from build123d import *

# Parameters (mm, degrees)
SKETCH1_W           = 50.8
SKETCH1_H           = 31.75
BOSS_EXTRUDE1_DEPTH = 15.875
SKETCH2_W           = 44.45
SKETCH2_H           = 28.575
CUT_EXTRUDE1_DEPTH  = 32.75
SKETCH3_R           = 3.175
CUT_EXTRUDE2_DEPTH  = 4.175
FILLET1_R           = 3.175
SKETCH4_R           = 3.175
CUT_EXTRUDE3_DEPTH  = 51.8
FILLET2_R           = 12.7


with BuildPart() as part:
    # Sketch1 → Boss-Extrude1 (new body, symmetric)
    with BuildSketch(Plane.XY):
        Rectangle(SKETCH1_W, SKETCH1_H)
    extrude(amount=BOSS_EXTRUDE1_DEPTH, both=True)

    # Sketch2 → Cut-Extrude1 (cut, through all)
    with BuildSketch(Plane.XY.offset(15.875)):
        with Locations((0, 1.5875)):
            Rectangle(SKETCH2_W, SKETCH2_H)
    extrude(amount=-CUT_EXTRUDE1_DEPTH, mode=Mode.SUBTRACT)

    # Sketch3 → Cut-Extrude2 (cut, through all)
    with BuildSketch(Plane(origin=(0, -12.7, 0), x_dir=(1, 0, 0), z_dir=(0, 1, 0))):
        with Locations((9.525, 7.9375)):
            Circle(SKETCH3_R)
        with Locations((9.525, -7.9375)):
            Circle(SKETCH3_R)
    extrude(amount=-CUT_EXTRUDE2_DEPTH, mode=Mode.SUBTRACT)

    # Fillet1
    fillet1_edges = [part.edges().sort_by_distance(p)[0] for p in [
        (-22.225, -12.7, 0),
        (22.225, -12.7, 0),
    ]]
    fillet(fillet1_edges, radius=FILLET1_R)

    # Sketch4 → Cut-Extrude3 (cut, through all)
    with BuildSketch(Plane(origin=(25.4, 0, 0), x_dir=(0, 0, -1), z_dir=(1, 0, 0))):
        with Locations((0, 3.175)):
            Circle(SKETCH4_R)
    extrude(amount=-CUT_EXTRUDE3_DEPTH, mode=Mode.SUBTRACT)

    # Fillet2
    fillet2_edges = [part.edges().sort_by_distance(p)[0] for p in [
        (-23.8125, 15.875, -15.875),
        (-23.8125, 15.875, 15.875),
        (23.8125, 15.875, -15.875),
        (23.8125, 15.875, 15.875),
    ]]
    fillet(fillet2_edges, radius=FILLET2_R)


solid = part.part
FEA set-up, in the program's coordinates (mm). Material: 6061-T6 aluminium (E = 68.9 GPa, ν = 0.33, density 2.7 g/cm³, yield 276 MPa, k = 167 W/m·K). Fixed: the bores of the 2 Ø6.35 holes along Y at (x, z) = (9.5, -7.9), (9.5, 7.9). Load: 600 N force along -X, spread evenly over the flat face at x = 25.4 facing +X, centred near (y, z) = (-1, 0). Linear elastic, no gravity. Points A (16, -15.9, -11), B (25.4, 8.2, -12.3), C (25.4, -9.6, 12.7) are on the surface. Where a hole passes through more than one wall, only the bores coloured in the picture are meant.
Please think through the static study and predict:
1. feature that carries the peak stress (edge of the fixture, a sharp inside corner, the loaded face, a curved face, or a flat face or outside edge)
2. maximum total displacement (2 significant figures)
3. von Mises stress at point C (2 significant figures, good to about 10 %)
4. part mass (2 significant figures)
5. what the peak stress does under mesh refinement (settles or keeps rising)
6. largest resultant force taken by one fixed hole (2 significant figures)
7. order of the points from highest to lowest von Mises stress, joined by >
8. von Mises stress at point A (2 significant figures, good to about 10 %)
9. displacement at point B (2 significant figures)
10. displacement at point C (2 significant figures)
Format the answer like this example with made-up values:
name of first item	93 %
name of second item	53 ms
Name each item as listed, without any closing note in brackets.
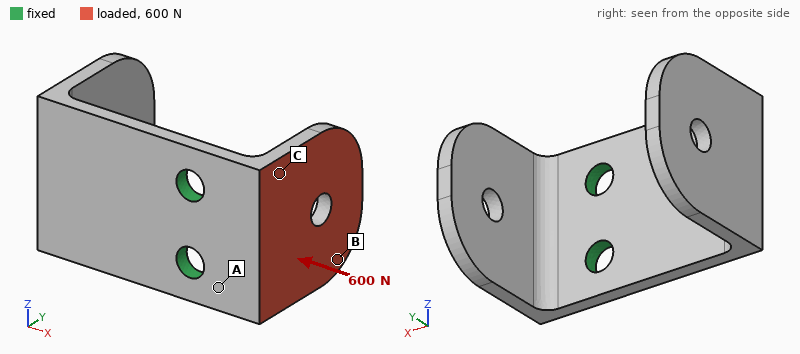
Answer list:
feature that carries the peak stress	edge of the fixture
maximum total displacement	0.62 mm
von Mises stress at point C	90 MPa
part mass	27 g
what the peak stress does under mesh refinement	keeps rising
largest resultant force taken by one fixed hole	310 N
order of the points from highest to lowest von Mises stress, joined by >	A > C > B
von Mises stress at point A	130 MPa
displacement at point B	0.44 mm
displacement at point C	0.13 mm
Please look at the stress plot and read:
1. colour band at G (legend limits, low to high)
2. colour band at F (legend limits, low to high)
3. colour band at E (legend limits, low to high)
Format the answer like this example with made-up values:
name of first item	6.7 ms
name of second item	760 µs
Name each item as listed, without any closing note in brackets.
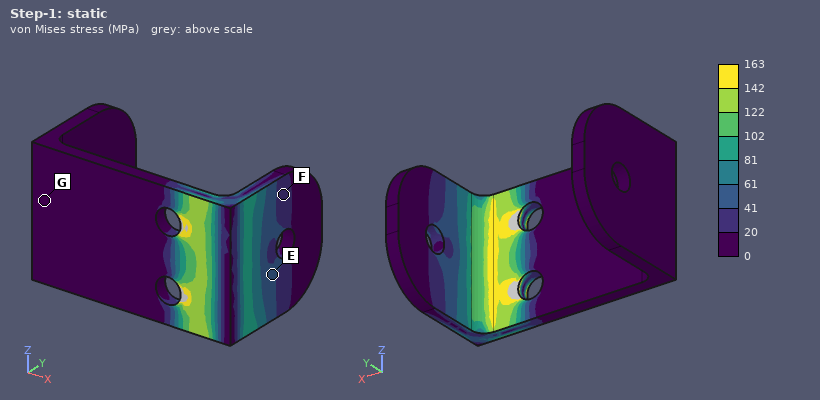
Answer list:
colour band at G	0 to 20 MPa
colour band at F	20 to 41 MPa
colour band at E	41 to 61 MPa
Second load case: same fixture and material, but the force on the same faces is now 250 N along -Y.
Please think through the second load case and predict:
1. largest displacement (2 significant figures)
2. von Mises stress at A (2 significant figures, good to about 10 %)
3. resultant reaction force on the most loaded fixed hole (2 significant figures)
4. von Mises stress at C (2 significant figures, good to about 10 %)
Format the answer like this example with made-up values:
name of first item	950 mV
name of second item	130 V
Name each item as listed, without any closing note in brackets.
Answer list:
largest displacement	0.13 mm
von Mises stress at A	40 MPa
resultant reaction force on the most loaded fixed hole	130 N
von Mises stress at C	7.0 MPa
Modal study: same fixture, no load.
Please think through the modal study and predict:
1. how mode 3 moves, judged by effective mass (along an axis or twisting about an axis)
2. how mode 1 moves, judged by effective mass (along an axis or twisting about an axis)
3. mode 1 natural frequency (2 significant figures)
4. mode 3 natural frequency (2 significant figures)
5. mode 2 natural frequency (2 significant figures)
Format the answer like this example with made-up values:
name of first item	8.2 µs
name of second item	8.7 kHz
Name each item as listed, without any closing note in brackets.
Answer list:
how mode 3 moves, judged by effective mass	along X
how mode 1 moves, judged by effective mass	along Y
mode 1 natural frequency	1000 Hz
mode 3 natural frequency	2200 Hz
mode 2 natural frequency	2000 Hz
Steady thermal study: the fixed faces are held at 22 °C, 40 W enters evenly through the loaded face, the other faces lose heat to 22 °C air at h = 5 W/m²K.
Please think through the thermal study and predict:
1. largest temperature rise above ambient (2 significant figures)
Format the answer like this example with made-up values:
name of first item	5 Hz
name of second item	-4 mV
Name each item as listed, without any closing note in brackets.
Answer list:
largest temperature rise above ambient	58 K
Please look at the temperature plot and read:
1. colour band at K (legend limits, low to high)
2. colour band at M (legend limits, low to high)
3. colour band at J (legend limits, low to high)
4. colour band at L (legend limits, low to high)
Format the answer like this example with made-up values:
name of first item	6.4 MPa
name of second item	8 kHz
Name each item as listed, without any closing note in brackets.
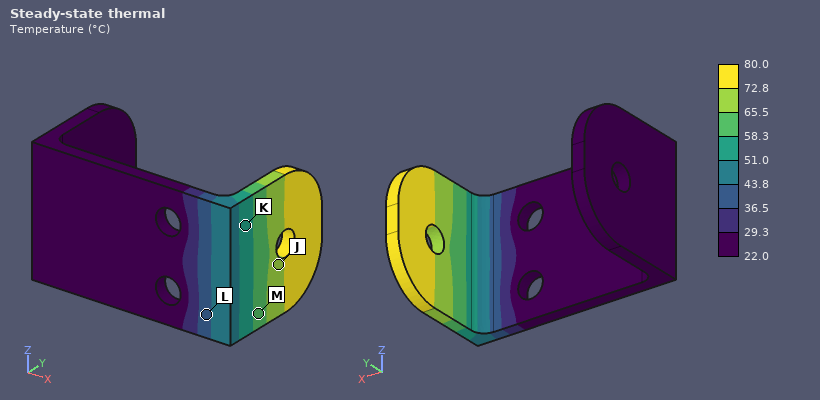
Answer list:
colour band at K	51.0 to 58.3 °C
colour band at M	58.3 to 65.5 °C
colour band at J	65.5 to 72.8 °C
colour band at L	36.5 to 43.8 °C
